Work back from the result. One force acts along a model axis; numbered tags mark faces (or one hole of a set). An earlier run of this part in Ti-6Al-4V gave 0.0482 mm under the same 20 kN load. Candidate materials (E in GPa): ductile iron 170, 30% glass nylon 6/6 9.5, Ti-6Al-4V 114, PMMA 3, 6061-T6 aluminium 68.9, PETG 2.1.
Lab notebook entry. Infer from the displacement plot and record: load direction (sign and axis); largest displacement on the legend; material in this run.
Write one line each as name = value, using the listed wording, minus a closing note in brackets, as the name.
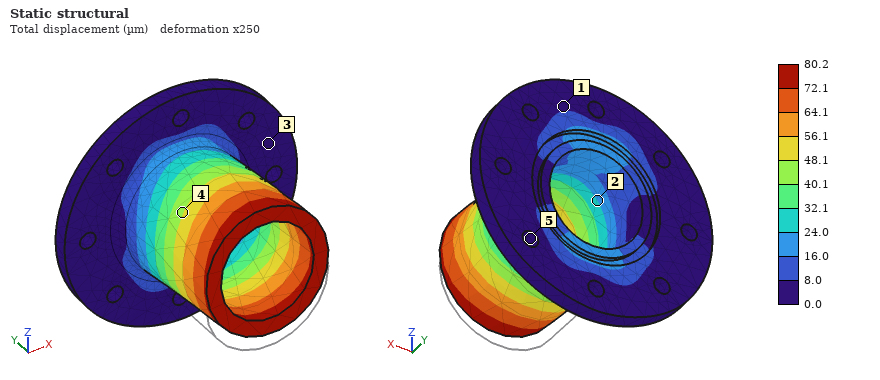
load direction = +Z
largest displacement on the legend = 80.2 µm
material in this run = 6061-T6 aluminium
